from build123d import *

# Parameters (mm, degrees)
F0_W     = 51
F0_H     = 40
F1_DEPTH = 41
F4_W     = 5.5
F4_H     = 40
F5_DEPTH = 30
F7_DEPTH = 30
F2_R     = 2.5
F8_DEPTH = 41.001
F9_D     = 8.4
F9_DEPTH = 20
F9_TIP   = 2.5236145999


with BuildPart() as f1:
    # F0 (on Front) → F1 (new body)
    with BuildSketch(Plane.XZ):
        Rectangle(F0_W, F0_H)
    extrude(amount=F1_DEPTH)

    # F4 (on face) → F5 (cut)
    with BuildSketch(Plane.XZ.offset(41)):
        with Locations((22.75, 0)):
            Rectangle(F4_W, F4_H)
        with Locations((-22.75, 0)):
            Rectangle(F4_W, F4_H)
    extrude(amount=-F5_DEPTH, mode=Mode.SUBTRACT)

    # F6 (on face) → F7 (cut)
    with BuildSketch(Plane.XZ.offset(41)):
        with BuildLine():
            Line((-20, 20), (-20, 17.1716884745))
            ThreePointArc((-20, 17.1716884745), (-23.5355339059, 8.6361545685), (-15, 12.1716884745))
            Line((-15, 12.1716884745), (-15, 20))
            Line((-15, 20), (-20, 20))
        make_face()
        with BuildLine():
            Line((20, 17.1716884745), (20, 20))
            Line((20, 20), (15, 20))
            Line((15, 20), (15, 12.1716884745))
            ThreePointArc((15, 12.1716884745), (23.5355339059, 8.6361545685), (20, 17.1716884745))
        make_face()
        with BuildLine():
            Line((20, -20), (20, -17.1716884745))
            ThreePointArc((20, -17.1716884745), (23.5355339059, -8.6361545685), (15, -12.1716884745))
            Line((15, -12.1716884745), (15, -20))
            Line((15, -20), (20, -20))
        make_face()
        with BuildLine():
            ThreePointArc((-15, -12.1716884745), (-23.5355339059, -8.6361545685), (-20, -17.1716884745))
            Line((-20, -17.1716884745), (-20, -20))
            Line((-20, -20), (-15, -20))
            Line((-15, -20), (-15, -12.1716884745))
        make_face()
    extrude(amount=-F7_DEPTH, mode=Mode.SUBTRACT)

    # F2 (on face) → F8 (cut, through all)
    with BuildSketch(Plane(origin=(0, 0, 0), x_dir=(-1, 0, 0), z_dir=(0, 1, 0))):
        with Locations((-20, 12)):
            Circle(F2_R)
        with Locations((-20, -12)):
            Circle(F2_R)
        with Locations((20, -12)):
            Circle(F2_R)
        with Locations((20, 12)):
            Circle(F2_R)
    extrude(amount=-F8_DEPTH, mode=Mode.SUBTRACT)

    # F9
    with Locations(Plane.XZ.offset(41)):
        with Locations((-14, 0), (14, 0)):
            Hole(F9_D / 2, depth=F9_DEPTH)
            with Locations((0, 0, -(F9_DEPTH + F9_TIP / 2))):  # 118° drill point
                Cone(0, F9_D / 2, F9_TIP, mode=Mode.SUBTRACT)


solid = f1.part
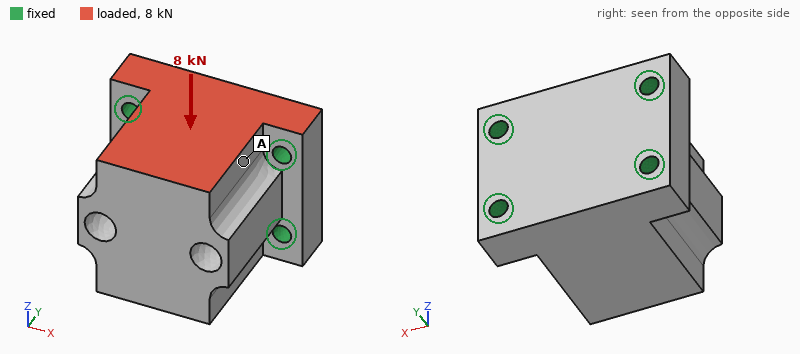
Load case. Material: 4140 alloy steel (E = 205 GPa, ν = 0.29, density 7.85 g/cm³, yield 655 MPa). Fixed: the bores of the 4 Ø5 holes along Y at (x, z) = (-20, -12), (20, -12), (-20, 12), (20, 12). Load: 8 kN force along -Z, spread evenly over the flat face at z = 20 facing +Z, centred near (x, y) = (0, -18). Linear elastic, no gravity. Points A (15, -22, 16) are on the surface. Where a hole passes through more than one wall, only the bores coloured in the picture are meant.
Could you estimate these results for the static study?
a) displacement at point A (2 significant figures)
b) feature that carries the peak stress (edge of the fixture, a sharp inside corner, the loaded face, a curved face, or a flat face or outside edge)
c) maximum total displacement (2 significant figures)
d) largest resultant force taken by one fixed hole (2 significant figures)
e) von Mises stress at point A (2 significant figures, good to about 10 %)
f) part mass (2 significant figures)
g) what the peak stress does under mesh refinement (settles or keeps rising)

3.9 µm
edge of the fixture
6.9 µm
3.0 kN
9.6 MPa
470 g
keeps rising
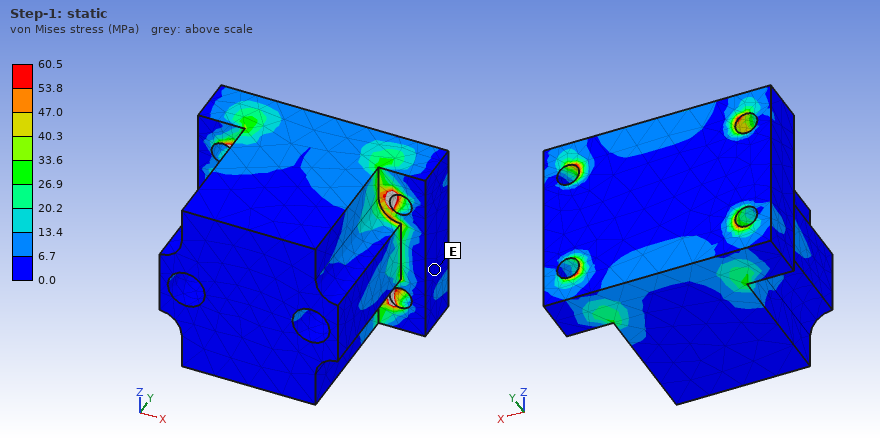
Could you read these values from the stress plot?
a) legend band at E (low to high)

0.0 to 6.7 MPa
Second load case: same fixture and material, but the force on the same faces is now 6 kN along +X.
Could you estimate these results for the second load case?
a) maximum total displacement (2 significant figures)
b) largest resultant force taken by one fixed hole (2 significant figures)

4.9 µm
2.9 kN
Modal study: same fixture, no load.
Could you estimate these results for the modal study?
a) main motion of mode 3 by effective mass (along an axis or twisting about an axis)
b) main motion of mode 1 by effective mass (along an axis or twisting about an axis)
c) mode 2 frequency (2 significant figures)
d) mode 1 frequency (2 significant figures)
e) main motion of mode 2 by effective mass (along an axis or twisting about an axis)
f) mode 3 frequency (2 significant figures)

along Y
along Z
13 kHz
9400 Hz
along X
18 kHz
